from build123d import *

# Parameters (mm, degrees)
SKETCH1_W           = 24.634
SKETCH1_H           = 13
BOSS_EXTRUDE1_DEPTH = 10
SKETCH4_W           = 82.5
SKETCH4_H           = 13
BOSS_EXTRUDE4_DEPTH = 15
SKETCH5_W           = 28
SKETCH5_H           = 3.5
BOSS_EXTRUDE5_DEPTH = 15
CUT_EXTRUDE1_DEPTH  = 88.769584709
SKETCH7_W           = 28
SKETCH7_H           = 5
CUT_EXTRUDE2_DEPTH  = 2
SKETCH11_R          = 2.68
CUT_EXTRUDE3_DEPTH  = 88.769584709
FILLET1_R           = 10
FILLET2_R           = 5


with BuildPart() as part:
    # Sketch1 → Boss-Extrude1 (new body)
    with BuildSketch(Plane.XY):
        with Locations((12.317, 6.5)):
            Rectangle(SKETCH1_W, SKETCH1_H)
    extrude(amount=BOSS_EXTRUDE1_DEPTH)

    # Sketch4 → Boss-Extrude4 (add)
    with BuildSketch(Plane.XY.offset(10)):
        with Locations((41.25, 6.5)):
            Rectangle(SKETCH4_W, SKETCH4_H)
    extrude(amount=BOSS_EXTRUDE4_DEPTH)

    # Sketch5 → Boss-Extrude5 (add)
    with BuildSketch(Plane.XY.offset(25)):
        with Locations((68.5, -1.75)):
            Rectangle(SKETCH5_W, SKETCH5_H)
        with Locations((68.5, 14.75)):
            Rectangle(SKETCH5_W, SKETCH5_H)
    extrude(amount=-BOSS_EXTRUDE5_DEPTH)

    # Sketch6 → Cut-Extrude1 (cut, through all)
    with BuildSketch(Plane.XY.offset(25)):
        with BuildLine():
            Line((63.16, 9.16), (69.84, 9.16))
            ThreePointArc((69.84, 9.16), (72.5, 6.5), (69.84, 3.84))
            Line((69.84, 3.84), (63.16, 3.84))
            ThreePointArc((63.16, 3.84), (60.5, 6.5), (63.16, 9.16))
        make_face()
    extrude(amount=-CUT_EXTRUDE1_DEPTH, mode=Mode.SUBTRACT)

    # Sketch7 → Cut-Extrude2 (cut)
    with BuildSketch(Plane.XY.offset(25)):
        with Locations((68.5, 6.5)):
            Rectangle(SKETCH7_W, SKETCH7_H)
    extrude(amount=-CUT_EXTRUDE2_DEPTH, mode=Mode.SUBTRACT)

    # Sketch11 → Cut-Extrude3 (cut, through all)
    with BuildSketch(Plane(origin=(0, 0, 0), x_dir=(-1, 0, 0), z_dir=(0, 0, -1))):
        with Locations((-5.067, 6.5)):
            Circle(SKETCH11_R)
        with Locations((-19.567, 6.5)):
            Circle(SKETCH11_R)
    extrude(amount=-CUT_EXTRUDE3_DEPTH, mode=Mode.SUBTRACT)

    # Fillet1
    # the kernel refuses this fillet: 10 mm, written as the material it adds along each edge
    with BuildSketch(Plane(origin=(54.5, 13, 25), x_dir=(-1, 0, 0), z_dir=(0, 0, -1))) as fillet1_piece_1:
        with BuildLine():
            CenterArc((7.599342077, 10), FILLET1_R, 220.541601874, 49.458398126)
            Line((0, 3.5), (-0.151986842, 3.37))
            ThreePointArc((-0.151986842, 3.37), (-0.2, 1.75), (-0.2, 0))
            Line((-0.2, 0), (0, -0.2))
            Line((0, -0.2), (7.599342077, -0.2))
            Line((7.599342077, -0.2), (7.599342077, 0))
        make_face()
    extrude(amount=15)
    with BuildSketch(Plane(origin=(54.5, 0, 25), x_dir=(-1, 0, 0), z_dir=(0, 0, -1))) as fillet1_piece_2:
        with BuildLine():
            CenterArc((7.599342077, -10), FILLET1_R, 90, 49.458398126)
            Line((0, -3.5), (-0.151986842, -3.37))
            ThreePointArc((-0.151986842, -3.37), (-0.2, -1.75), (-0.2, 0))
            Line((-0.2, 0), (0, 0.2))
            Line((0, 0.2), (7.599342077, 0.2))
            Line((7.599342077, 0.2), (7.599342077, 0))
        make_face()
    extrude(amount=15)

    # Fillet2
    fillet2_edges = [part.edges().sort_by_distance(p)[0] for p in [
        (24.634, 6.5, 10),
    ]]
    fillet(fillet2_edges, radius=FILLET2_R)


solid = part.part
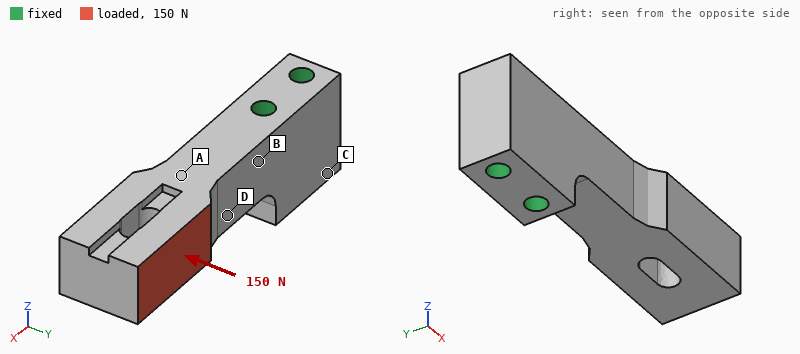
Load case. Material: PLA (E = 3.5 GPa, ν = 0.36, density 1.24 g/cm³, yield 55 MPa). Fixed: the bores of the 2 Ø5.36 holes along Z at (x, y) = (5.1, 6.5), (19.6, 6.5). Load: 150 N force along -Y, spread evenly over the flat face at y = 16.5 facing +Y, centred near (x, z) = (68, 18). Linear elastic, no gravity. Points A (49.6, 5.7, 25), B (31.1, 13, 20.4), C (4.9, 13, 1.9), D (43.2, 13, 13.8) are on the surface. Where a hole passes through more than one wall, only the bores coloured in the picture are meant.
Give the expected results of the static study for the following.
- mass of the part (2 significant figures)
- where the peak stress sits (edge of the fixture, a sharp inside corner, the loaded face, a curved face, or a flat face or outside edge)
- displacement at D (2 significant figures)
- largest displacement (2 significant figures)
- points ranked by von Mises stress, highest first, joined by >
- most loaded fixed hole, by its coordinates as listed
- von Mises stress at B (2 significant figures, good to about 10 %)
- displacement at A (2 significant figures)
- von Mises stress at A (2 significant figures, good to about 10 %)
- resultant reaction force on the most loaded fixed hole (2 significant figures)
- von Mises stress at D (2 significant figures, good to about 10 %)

25 g
a curved face
0.23 mm
0.92 mm
B > D > A > C
(19.6, 6.5)
13 MPa
0.30 mm
3.9 MPa
310 N
9.5 MPa
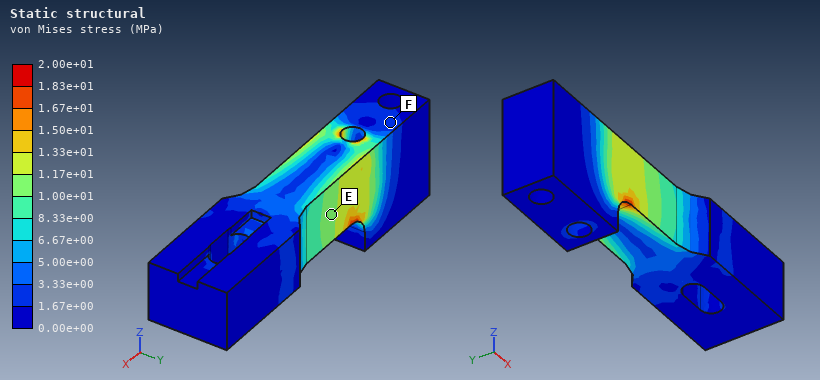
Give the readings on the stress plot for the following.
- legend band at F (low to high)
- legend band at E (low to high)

1.67e+00 to 3.33e+00 MPa
1.00e+01 to 1.17e+01 MPa
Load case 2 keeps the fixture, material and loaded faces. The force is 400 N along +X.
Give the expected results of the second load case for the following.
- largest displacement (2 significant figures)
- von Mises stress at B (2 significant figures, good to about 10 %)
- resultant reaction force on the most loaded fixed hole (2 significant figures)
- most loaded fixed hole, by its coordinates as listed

0.72 mm
11 MPa
380 N
(19.6, 6.5)
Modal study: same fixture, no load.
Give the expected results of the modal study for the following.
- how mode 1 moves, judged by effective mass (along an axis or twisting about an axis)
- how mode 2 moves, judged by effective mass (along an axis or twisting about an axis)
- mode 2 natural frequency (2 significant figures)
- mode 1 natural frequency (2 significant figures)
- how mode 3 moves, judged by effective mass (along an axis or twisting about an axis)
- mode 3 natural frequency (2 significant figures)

along Y
along Z
940 Hz
730 Hz
twisting about X
2800 Hz
